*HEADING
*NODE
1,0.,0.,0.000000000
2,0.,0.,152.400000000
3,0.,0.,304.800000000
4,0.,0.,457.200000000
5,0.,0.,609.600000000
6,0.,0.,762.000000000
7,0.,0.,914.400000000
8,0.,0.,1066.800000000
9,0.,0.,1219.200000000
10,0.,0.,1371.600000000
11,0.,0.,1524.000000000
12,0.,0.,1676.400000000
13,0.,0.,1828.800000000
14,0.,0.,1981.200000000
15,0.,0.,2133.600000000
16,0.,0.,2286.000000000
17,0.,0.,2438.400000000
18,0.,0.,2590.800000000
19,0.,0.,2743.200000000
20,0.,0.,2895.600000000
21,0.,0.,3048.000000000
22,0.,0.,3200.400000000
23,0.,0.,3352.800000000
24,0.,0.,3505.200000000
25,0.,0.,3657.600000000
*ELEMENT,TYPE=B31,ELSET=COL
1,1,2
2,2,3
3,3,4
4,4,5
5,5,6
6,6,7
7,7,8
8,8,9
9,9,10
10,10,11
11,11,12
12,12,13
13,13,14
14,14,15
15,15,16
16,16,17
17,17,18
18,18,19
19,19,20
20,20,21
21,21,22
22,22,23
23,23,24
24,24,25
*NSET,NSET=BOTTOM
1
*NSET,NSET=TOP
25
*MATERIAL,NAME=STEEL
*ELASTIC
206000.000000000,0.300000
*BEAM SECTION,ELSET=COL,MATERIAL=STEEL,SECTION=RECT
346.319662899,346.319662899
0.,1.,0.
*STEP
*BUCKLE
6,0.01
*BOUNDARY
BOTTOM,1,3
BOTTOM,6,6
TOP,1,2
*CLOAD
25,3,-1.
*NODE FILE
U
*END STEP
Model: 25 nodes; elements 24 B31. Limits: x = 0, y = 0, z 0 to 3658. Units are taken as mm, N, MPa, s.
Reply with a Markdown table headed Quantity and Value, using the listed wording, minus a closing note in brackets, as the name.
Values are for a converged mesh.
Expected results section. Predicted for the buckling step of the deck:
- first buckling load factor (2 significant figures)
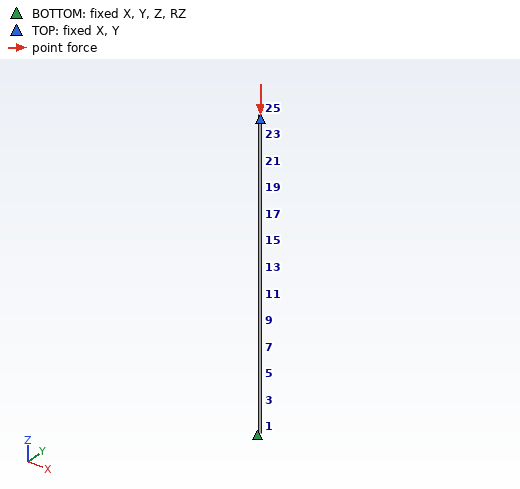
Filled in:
| Quantity | Value |
|---|---|
| first buckling load factor | 1.8e+08 |
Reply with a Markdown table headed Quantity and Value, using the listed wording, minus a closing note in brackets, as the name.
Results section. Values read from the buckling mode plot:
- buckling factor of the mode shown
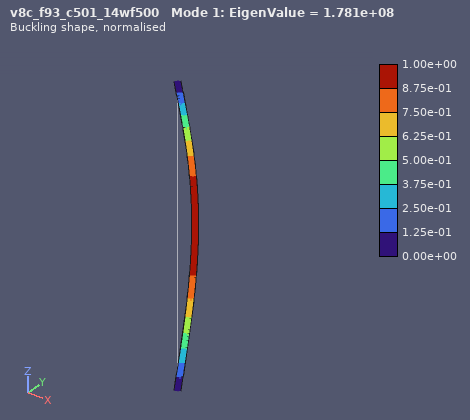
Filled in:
| Quantity | Value |
|---|---|
| buckling factor of the mode shown | 1.781e+08 |
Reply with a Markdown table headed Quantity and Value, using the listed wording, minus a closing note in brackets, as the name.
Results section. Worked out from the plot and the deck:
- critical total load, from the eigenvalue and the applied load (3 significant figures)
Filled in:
| Quantity | Value |
|---|---|
| critical total load, from the eigenvalue and the applied load | 1.78e+08 N |
